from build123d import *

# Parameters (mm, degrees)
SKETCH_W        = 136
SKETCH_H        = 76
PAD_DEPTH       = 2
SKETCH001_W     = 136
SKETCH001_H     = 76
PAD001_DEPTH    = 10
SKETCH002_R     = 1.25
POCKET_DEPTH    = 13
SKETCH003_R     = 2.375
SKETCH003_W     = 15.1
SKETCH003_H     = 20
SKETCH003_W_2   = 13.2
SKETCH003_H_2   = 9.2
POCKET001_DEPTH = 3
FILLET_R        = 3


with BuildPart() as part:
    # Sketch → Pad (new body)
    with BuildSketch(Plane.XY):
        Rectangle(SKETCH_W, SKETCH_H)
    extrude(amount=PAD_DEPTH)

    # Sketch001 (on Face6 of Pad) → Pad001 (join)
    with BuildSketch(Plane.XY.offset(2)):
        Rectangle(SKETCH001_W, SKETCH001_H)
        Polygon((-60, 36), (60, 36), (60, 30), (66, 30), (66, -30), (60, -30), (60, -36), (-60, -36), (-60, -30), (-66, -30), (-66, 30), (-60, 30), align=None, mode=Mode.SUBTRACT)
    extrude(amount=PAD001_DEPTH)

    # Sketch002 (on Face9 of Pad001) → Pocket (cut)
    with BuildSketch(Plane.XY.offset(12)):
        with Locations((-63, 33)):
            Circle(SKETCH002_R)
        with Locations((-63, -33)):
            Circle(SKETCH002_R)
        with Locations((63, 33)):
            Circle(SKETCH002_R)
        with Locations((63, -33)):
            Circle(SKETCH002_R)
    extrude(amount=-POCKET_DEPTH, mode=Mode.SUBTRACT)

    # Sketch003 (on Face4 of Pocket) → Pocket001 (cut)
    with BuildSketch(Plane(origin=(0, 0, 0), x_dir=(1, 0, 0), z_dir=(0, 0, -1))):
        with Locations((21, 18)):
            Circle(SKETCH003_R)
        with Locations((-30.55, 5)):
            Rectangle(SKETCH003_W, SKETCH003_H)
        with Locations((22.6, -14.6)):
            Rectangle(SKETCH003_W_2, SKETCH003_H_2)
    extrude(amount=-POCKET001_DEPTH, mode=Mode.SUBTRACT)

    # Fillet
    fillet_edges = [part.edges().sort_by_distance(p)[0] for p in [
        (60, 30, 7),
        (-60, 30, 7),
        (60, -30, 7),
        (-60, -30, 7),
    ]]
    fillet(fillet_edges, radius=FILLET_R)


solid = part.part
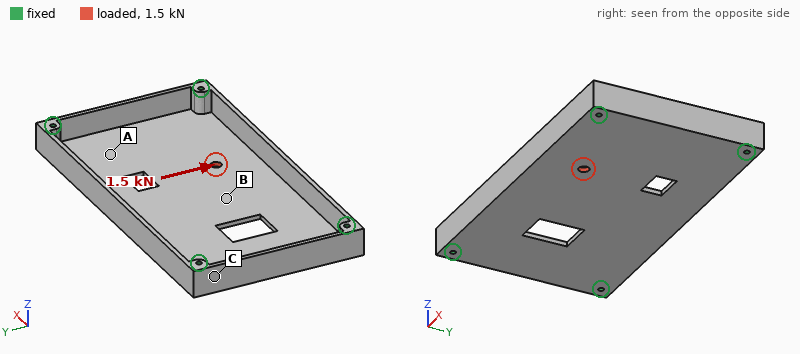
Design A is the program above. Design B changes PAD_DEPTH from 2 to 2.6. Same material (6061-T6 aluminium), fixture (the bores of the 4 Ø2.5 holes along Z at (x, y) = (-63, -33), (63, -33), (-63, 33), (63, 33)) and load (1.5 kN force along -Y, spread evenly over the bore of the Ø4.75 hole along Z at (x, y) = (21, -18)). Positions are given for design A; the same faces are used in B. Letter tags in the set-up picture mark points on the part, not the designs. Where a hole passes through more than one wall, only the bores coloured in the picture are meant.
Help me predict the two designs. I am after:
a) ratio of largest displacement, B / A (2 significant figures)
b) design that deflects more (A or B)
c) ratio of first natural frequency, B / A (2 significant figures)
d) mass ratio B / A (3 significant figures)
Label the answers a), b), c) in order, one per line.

a) 0.81
b) A
c) 1.2
d) 1.18
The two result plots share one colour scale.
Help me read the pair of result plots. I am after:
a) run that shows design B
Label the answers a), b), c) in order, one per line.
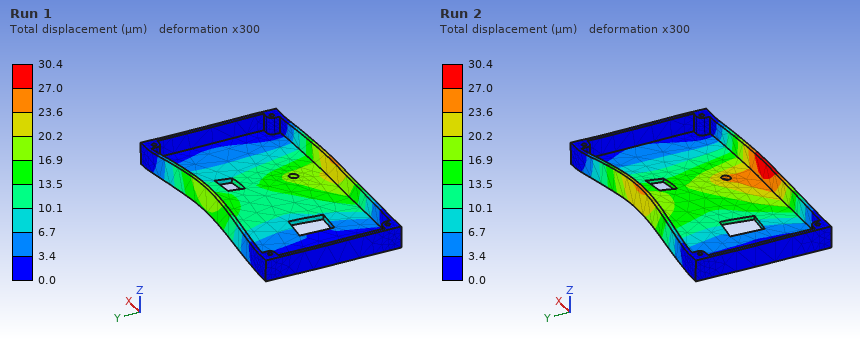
a) Run 1
